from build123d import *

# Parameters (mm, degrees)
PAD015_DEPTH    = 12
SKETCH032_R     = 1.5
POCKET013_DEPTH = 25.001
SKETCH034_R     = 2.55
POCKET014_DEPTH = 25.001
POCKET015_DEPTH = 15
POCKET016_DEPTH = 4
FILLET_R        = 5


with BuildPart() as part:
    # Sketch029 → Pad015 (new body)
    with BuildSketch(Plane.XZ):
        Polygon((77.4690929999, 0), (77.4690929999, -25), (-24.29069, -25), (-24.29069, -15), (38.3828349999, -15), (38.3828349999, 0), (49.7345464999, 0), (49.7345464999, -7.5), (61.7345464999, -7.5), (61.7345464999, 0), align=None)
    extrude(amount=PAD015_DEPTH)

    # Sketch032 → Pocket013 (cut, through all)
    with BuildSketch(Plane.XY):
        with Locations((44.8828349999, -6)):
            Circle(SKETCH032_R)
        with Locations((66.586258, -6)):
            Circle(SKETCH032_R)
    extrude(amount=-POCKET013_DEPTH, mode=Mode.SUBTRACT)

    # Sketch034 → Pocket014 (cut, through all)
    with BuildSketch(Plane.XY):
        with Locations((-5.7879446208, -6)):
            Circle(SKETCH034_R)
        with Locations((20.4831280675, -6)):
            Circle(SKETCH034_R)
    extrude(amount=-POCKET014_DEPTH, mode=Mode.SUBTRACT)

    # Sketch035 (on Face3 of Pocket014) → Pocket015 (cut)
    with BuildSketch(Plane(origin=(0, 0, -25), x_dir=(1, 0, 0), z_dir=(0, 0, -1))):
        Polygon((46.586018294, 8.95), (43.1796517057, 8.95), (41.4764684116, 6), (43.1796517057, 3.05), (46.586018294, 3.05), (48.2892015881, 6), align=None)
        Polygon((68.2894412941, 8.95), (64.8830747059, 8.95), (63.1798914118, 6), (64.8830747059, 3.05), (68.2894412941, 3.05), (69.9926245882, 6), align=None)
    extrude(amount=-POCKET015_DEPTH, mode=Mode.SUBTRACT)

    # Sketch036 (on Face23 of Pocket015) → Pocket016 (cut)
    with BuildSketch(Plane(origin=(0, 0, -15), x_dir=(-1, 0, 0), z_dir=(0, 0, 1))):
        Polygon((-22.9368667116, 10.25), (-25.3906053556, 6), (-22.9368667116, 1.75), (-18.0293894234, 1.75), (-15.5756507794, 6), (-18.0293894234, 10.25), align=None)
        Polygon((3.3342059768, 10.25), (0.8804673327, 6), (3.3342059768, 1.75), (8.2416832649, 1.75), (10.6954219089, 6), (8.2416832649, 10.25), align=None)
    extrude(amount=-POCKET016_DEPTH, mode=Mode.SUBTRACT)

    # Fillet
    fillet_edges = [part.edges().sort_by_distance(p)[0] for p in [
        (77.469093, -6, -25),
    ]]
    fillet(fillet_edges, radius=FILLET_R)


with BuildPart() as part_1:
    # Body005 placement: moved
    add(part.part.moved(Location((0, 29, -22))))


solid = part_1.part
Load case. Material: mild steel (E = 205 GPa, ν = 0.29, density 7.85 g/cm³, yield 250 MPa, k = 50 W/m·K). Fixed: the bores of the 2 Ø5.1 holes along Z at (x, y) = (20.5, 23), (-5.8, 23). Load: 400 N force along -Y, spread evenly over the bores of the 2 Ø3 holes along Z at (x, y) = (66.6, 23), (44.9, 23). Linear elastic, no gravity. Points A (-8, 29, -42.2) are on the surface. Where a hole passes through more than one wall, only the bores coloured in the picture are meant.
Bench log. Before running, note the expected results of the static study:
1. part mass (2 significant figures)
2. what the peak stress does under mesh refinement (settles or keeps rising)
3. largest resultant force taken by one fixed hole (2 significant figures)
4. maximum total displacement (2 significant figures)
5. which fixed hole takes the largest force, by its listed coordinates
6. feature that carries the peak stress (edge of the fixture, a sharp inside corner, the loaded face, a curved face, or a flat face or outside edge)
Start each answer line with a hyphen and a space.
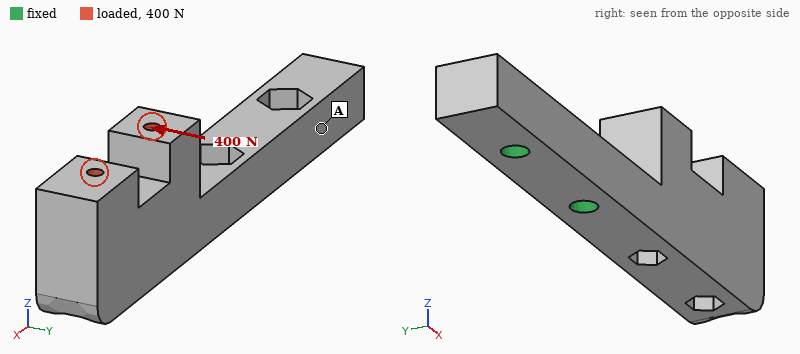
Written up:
- 130 g
- keeps rising
- 610 N
- 71 µm
- (20.5, 23)
- edge of the fixture
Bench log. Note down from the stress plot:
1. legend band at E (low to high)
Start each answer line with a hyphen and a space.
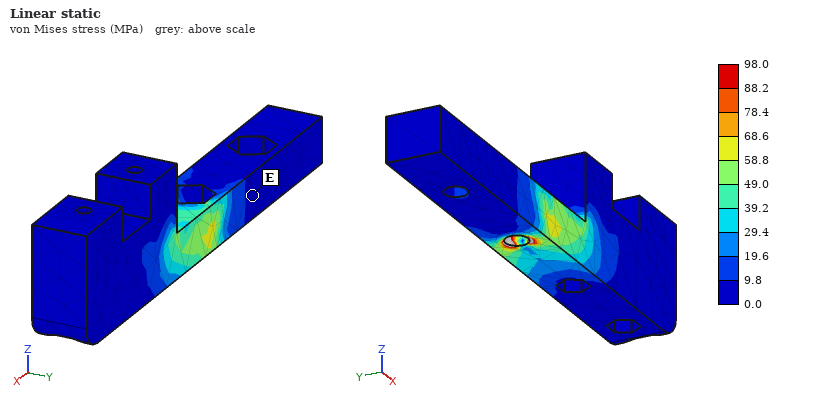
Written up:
- 0.0 to 9.8 MPa
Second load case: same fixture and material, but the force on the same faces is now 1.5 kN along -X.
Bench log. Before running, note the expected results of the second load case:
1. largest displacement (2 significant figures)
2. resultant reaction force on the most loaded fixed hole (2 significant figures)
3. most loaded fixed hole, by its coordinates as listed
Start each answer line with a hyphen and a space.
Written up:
- 0.19 mm
- 930 N
- (20.5, 23)
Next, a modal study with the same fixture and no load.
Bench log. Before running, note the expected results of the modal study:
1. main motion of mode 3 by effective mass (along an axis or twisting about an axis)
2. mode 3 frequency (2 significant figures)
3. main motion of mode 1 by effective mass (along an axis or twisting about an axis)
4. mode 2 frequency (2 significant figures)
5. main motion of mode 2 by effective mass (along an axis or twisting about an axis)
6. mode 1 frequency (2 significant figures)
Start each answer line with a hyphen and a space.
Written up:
- twisting about X
- 5200 Hz
- along Z
- 1800 Hz
- along Y
- 1400 Hz
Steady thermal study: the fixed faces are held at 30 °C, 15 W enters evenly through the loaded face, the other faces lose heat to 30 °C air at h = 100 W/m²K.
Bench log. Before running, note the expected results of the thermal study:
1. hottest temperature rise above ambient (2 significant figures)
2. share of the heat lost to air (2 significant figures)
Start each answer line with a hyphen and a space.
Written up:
- 34 K
- 70 %
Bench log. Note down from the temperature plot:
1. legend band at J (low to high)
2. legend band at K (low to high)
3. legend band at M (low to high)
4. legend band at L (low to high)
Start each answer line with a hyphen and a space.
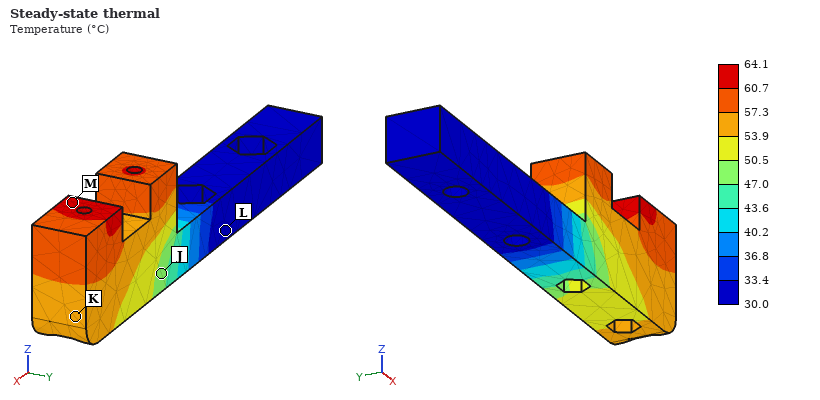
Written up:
- 47.0 to 50.5 °C
- 53.9 to 57.3 °C
- 60.7 to 64.1 °C
- 30.0 to 33.4 °C
